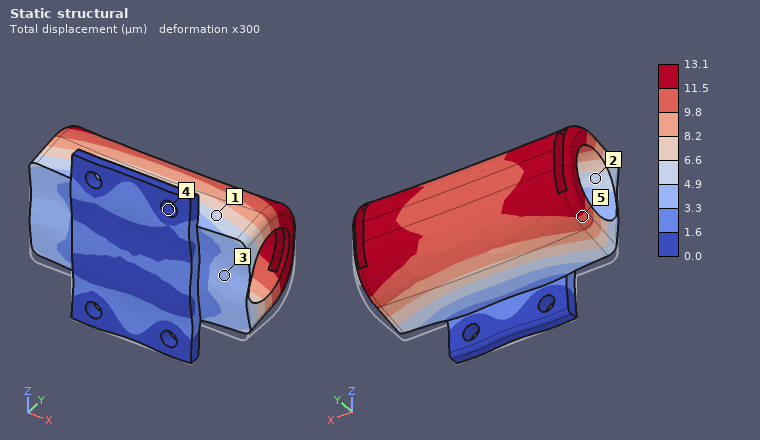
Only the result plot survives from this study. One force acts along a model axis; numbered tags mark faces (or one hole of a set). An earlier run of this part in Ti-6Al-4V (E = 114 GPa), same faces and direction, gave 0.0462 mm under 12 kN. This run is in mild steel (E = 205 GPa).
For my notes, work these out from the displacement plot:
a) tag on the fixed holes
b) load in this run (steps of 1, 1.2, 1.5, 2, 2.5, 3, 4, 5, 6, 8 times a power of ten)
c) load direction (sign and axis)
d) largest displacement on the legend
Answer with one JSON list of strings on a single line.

["4", "6 kN", "+Z", "13.1 µm"]
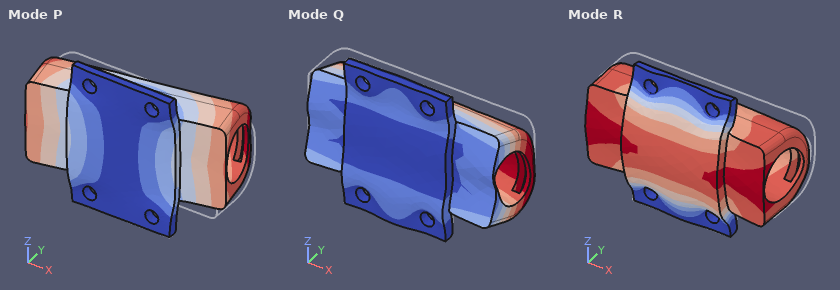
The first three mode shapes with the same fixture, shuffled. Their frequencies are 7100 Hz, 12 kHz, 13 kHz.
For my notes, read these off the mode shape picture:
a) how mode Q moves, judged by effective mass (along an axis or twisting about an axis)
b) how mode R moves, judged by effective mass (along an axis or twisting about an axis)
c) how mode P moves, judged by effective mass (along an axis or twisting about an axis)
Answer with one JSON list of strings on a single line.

["along Z", "along Y", "along X"]
